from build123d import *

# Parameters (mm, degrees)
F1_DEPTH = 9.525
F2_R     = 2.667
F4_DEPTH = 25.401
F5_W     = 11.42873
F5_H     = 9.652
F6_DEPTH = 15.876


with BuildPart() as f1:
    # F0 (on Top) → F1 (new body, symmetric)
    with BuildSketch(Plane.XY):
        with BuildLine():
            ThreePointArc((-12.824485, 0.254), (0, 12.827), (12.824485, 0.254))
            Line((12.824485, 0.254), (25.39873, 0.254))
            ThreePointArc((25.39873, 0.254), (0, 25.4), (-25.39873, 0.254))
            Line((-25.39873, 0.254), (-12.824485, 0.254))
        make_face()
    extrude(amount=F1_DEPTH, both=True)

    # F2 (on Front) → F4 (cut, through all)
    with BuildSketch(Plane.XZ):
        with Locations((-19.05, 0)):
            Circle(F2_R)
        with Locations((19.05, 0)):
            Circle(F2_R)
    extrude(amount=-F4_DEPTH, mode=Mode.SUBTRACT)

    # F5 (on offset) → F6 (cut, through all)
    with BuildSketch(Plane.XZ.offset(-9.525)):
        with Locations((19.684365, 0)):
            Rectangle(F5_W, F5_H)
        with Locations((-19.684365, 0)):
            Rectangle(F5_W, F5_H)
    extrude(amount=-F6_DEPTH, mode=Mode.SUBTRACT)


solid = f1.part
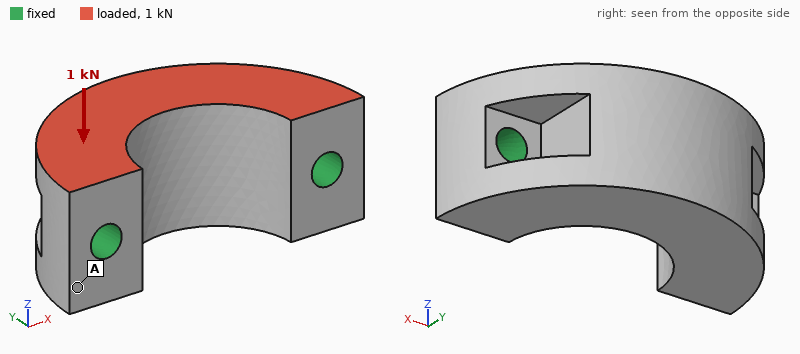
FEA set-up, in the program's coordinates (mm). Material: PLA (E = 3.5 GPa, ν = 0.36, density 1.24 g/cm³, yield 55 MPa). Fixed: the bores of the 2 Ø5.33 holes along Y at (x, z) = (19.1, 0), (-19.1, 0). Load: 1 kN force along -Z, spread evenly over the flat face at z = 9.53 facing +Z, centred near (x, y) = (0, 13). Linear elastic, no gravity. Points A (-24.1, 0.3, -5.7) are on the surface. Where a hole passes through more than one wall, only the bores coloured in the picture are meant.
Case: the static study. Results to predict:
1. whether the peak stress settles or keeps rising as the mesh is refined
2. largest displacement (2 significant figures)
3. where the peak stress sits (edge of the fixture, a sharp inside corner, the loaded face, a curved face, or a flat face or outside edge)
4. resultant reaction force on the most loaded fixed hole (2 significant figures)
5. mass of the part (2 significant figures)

keeps rising
0.15 mm
edge of the fixture
500 N
16 g
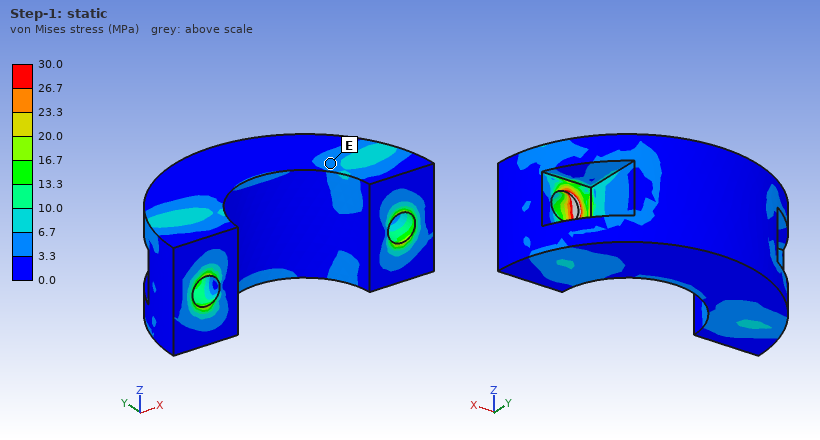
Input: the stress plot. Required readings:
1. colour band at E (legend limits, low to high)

3.3 to 6.7 MPa
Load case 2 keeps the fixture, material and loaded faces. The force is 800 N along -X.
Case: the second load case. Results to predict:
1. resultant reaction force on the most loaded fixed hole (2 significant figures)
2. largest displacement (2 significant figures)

440 N
52 µm
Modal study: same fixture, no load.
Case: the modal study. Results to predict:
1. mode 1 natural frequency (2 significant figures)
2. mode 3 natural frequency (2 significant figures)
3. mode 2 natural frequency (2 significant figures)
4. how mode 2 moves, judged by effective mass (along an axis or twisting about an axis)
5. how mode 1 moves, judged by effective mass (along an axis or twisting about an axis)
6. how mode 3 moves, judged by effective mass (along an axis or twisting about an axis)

3900 Hz
9200 Hz
8500 Hz
along X
along Z
along Y
